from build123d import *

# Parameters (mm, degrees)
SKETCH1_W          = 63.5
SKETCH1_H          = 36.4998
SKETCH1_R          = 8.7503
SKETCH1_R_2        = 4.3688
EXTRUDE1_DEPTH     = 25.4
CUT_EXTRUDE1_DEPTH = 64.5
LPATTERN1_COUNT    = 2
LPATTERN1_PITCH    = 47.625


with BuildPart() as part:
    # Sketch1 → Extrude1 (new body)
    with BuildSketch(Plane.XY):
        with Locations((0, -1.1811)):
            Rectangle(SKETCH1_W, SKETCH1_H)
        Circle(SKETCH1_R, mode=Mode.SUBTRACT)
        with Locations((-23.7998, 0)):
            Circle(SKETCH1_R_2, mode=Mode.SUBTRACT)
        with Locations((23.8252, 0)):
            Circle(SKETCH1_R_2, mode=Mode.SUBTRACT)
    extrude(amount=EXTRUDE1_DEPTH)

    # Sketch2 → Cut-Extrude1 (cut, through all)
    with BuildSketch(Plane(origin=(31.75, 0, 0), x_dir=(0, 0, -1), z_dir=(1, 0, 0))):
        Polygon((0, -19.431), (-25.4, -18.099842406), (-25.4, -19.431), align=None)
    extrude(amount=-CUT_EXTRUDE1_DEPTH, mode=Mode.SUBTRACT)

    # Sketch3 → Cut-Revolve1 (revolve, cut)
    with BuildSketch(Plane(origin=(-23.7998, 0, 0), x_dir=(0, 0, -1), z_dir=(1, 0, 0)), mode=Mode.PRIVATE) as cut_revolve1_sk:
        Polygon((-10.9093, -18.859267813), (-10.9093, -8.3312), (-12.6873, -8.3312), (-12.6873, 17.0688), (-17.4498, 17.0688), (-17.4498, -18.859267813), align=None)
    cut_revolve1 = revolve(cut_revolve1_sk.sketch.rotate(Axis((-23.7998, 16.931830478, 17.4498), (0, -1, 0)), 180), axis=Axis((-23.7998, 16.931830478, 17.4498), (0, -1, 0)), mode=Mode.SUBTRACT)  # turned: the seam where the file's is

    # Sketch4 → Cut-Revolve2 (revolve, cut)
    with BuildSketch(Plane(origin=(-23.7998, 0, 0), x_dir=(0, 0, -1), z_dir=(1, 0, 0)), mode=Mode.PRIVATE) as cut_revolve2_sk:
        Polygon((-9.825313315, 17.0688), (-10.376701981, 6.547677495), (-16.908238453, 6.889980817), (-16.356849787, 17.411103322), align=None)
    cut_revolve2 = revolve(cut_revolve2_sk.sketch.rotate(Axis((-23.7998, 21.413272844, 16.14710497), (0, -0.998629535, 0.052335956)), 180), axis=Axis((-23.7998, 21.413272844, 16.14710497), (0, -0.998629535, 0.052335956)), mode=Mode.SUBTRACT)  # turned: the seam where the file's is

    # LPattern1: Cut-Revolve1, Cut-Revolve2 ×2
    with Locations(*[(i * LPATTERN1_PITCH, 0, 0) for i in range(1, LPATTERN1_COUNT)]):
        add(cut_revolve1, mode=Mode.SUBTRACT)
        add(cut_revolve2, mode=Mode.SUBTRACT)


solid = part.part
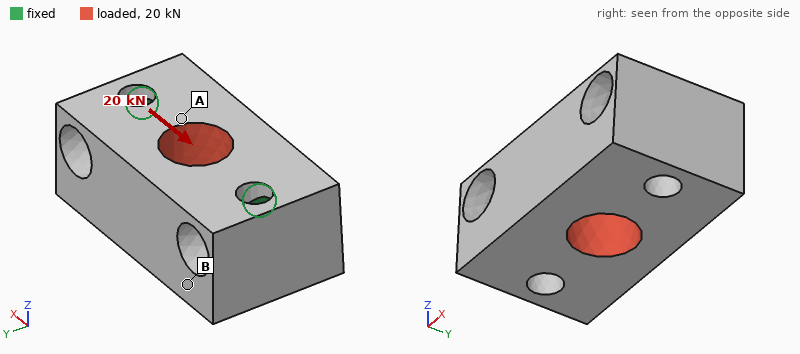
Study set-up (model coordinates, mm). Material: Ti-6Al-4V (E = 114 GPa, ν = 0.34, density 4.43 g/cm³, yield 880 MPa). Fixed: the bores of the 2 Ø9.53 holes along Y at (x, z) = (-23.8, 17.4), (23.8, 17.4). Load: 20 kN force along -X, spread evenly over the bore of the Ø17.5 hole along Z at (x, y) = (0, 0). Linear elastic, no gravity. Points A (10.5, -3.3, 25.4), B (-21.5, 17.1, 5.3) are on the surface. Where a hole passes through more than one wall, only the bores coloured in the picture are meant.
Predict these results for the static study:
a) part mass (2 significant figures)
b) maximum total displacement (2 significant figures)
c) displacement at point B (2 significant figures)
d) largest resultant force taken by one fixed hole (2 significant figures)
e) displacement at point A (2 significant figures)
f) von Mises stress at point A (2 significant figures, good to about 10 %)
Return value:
190 g
6.0 µm
4.5 µm
10 kN
2.1 µm
21 MPa
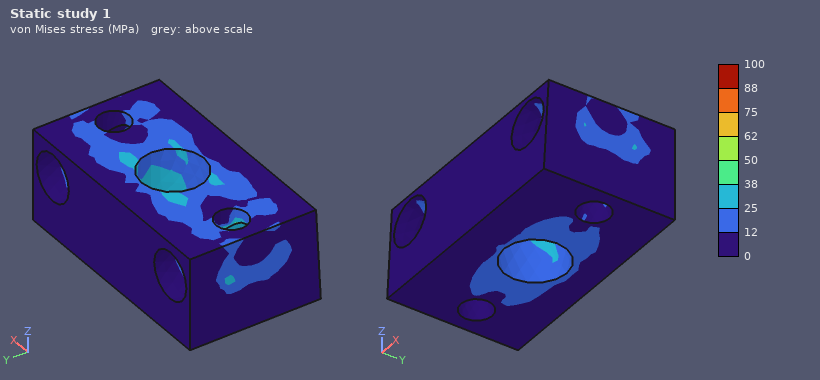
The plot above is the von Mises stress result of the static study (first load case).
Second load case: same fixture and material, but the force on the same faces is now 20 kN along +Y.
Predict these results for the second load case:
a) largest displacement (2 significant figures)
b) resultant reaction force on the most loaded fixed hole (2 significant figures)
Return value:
19 µm
10 kN
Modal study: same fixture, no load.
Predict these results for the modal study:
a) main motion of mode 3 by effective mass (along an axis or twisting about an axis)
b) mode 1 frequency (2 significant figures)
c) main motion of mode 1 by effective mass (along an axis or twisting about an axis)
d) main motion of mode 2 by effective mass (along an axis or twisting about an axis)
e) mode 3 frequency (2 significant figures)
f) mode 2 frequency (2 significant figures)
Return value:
twisting about Z
13 kHz
along Y
along Z
23 kHz
20 kHz
